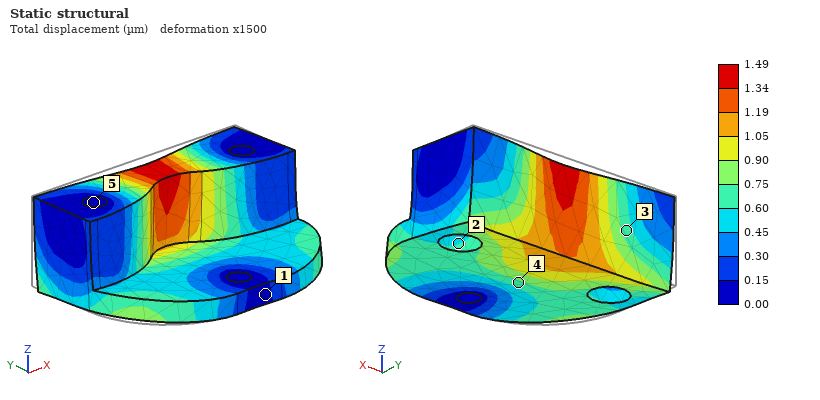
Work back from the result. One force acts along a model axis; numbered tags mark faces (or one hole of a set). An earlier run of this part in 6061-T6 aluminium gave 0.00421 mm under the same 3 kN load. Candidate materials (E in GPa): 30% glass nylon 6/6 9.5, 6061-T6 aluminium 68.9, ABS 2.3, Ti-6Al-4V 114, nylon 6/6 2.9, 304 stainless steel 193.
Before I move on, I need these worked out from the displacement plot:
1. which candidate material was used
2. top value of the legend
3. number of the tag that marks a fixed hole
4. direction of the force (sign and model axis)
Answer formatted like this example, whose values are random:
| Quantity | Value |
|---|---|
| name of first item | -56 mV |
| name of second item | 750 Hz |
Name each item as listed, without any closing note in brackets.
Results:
| Quantity | Value |
|---|---|
| which candidate material was used | 304 stainless steel |
| top value of the legend | 1.49 µm |
| number of the tag that marks a fixed hole | 5 |
| direction of the force | -Y |
